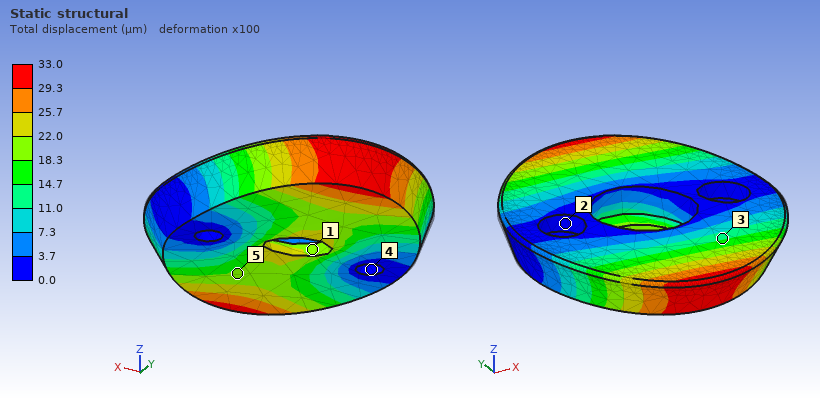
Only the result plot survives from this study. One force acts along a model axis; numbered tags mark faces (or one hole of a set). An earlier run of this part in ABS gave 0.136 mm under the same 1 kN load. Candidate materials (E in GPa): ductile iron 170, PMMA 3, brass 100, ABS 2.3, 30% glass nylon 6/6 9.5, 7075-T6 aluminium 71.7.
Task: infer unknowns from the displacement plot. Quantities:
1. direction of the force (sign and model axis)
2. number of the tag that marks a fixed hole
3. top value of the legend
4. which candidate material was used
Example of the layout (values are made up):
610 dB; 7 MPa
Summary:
+Y; 4; 33.0 µm; 30% glass nylon 6/6
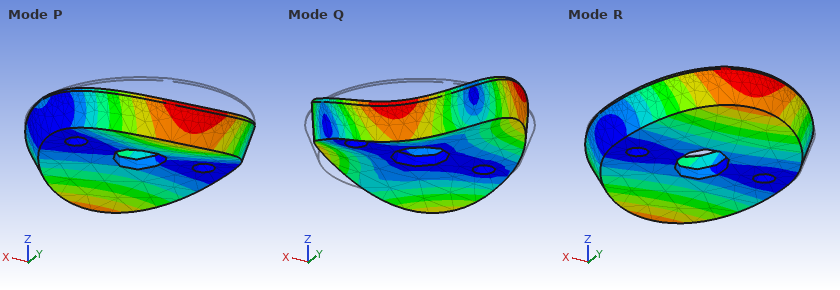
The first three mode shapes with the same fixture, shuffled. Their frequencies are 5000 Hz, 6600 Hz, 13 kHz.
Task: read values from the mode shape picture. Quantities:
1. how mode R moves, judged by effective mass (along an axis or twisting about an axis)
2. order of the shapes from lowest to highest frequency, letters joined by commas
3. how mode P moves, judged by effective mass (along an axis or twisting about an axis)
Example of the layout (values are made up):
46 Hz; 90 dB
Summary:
twisting about X; R, P, Q; along Z
